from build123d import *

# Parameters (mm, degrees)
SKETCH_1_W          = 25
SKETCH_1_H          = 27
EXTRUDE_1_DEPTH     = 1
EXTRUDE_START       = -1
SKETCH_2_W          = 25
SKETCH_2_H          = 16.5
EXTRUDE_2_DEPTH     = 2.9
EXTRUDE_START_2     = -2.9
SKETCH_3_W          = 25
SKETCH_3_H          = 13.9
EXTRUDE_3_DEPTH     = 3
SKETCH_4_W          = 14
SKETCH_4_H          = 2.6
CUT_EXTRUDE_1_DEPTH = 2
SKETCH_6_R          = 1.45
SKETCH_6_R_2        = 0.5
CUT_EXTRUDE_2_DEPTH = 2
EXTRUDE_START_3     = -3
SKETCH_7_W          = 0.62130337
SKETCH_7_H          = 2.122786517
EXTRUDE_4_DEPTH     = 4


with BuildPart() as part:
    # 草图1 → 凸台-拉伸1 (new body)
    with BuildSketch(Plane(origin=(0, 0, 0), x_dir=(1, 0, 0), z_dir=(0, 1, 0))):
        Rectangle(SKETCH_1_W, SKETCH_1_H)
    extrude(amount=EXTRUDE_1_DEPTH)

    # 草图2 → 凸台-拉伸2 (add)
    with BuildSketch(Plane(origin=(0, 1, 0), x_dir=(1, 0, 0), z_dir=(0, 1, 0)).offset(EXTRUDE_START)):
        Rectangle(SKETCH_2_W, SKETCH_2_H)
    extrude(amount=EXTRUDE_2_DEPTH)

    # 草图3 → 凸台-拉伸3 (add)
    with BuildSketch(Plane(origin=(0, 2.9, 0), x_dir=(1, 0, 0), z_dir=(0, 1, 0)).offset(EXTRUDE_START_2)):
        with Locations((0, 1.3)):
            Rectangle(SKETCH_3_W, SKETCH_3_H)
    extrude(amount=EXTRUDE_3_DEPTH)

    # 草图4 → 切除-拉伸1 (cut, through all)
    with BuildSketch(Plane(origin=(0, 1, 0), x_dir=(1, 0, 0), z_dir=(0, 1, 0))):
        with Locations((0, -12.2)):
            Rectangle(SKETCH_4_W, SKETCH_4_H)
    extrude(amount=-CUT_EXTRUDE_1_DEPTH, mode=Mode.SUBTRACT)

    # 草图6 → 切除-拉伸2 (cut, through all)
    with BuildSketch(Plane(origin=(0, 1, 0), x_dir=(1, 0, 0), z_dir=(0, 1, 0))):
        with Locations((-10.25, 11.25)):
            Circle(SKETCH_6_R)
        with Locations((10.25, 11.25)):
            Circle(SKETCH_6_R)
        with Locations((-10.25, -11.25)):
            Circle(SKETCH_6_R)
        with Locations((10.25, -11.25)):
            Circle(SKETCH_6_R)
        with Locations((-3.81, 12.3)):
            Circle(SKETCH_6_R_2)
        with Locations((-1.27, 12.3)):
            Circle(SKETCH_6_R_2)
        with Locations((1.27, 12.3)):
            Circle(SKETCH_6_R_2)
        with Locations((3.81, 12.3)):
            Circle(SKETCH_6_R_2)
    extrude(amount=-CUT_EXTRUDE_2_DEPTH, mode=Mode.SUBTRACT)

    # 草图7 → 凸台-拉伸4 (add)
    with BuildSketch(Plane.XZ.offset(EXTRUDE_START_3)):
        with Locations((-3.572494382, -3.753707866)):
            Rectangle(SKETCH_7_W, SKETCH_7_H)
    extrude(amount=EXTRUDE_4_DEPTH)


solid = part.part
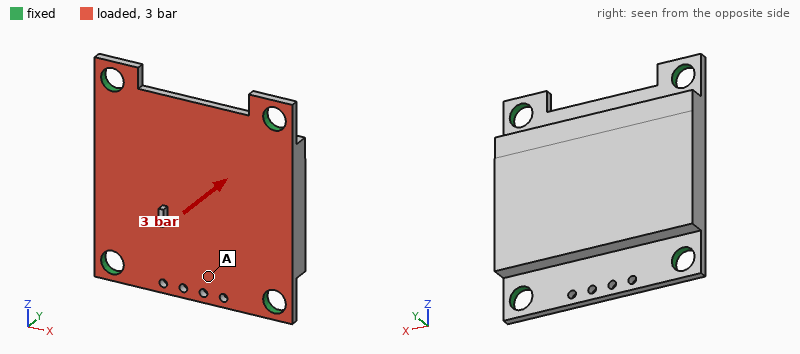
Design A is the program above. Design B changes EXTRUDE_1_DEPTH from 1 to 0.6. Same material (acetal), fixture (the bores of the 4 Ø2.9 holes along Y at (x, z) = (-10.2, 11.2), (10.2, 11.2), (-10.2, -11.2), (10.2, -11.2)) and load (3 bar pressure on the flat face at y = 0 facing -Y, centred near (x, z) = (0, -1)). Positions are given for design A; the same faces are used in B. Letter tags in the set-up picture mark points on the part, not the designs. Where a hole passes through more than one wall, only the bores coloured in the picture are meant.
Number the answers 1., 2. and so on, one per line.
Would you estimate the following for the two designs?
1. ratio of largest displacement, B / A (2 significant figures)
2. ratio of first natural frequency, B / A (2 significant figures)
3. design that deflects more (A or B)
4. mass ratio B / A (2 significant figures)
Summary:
1. 2.8
2. 0.77
3. B
4. 0.94
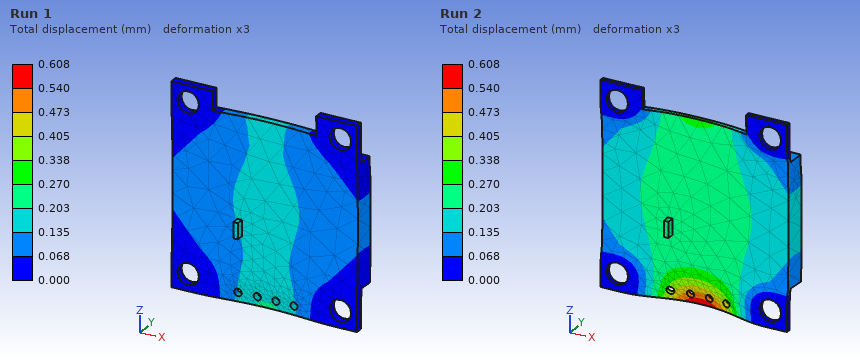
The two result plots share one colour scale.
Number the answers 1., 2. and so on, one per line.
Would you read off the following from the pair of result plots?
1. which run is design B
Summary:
1. Run 2
